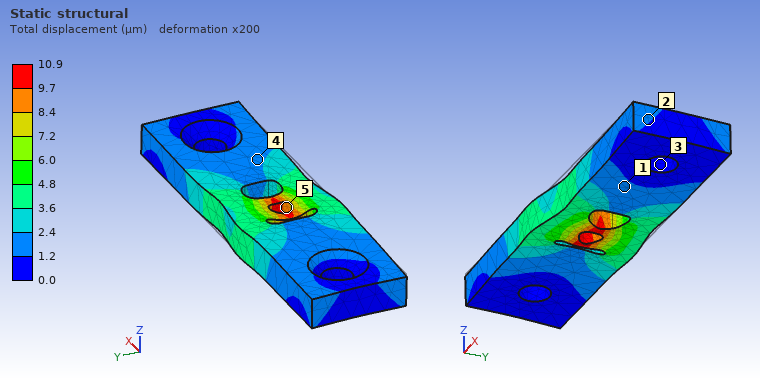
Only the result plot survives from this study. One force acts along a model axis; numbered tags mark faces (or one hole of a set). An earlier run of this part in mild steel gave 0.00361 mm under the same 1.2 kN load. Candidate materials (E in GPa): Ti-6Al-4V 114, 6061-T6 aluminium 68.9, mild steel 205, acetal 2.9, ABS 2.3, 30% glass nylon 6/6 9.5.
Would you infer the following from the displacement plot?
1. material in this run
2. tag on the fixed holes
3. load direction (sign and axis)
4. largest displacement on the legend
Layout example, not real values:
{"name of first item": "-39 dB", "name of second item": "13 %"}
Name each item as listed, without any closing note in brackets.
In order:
{"material in this run": "6061-T6 aluminium", "tag on the fixed holes": "3", "load direction": "-X", "largest displacement on the legend": "10.9 µm"}
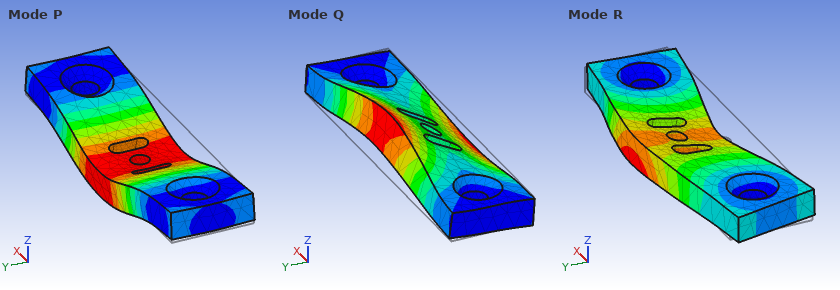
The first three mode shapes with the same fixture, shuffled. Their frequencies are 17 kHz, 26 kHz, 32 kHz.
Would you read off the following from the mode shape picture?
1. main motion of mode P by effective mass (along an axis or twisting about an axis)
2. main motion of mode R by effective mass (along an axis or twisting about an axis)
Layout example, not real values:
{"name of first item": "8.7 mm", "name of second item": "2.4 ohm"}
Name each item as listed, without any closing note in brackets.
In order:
{"main motion of mode P by effective mass": "along Z", "main motion of mode R by effective mass": "along Y"}
